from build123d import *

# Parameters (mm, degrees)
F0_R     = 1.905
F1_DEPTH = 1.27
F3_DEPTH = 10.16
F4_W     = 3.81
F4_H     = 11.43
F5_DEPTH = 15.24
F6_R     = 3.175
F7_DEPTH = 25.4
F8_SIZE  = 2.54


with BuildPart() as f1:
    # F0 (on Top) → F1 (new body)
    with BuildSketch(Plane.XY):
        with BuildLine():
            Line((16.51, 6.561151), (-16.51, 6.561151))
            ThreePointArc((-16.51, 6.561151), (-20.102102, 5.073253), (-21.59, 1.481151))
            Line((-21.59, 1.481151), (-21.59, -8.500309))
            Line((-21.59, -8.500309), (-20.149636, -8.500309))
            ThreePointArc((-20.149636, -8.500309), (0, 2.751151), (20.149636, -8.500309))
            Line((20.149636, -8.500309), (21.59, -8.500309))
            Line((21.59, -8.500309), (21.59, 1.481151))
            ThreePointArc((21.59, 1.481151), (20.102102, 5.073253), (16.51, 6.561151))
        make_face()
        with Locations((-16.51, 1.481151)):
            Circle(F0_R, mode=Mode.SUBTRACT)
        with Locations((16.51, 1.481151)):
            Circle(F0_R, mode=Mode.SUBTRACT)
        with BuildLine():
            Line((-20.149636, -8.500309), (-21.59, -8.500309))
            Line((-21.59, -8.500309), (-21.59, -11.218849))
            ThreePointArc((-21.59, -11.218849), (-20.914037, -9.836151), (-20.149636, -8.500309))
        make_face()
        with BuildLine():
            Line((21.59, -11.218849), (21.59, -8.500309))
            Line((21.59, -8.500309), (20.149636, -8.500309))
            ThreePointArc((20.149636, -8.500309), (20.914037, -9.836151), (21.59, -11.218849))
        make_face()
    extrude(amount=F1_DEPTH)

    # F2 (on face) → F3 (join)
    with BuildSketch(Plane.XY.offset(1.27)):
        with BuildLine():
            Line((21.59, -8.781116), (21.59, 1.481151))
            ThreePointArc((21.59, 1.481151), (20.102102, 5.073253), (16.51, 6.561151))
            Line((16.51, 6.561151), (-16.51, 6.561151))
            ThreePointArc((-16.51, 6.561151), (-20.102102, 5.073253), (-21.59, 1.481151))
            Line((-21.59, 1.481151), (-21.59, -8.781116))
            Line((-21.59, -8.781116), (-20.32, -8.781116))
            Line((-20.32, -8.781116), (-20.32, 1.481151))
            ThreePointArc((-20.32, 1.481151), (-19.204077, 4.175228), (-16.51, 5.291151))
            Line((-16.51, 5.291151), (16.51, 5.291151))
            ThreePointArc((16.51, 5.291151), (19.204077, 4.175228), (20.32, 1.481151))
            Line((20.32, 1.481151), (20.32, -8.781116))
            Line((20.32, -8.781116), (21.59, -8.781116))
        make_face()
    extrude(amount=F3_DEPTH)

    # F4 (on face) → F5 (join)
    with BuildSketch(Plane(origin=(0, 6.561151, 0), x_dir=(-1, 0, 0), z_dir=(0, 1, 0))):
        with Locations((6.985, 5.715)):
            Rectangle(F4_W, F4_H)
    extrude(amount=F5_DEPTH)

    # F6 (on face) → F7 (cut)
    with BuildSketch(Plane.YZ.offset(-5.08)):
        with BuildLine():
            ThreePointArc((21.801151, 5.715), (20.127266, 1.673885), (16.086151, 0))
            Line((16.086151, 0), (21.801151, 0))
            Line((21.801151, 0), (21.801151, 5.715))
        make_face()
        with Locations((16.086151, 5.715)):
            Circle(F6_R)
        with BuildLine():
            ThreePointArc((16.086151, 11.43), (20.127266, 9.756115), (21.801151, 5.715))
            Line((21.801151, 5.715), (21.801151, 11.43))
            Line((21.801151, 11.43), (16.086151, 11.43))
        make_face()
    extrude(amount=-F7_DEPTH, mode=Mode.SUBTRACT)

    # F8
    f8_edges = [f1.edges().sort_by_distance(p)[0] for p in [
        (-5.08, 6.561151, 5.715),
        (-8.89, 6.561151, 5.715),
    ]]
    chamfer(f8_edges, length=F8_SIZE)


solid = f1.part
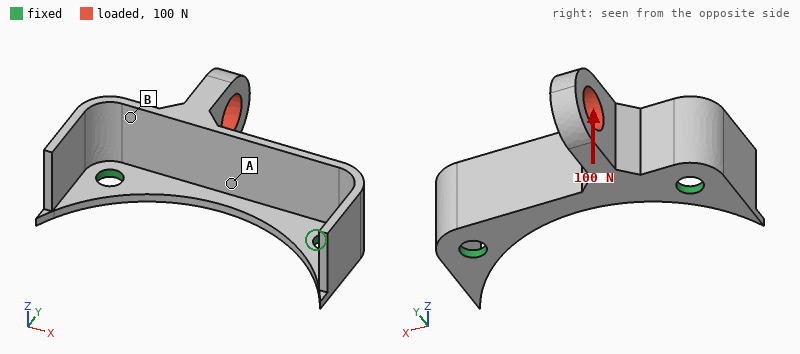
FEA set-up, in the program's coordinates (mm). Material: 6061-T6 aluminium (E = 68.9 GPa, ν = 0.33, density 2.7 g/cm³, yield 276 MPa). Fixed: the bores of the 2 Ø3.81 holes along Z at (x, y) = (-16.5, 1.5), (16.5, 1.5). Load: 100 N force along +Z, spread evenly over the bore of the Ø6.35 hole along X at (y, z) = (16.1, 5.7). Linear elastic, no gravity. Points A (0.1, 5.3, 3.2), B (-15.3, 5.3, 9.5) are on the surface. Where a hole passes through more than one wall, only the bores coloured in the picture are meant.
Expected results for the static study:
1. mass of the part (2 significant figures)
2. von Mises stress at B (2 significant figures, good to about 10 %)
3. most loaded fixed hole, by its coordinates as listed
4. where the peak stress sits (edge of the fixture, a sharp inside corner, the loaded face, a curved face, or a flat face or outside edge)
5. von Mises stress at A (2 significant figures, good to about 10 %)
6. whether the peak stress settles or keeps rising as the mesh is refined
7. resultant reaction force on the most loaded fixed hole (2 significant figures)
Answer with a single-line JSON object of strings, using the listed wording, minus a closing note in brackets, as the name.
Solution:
{"mass of the part": "4.9 g", "von Mises stress at B": "71 MPa", "most loaded fixed hole, by its coordinates as listed": "(-16.5, 1.5)", "where the peak stress sits": "edge of the fixture", "von Mises stress at A": "29 MPa", "whether the peak stress settles or keeps rising as the mesh is refined": "keeps rising", "resultant reaction force on the most loaded fixed hole": "78 N"}
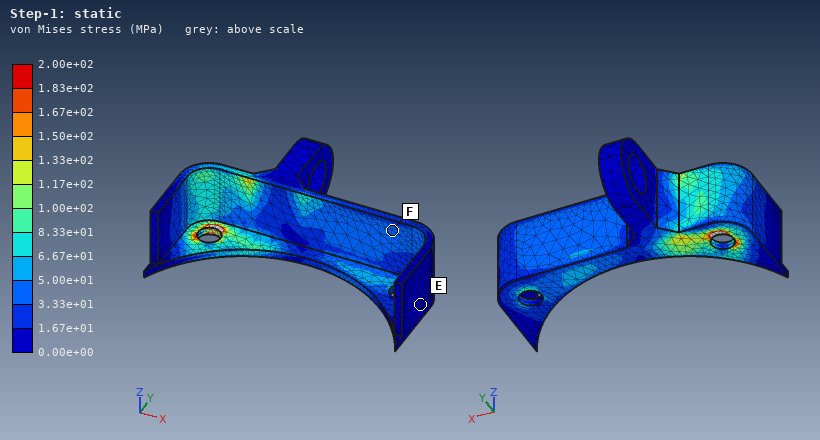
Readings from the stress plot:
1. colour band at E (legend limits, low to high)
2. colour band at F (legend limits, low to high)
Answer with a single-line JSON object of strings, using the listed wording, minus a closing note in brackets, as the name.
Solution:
{"colour band at E": "0.00e+00 to 1.67e+01 MPa", "colour band at F": "3.33e+01 to 5.00e+01 MPa"}
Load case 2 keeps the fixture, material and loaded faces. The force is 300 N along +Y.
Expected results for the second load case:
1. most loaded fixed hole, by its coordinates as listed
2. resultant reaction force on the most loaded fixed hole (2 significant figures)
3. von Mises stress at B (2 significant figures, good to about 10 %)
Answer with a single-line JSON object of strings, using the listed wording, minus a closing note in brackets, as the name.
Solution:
{"most loaded fixed hole, by its coordinates as listed": "(-16.5, 1.5)", "resultant reaction force on the most loaded fixed hole": "260 N", "von Mises stress at B": "99 MPa"}
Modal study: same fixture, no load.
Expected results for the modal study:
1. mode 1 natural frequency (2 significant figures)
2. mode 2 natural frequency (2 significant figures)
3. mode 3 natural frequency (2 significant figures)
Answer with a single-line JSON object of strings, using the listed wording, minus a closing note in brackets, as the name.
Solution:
{"mode 1 natural frequency": "3000 Hz", "mode 2 natural frequency": "8200 Hz", "mode 3 natural frequency": "9000 Hz"}
